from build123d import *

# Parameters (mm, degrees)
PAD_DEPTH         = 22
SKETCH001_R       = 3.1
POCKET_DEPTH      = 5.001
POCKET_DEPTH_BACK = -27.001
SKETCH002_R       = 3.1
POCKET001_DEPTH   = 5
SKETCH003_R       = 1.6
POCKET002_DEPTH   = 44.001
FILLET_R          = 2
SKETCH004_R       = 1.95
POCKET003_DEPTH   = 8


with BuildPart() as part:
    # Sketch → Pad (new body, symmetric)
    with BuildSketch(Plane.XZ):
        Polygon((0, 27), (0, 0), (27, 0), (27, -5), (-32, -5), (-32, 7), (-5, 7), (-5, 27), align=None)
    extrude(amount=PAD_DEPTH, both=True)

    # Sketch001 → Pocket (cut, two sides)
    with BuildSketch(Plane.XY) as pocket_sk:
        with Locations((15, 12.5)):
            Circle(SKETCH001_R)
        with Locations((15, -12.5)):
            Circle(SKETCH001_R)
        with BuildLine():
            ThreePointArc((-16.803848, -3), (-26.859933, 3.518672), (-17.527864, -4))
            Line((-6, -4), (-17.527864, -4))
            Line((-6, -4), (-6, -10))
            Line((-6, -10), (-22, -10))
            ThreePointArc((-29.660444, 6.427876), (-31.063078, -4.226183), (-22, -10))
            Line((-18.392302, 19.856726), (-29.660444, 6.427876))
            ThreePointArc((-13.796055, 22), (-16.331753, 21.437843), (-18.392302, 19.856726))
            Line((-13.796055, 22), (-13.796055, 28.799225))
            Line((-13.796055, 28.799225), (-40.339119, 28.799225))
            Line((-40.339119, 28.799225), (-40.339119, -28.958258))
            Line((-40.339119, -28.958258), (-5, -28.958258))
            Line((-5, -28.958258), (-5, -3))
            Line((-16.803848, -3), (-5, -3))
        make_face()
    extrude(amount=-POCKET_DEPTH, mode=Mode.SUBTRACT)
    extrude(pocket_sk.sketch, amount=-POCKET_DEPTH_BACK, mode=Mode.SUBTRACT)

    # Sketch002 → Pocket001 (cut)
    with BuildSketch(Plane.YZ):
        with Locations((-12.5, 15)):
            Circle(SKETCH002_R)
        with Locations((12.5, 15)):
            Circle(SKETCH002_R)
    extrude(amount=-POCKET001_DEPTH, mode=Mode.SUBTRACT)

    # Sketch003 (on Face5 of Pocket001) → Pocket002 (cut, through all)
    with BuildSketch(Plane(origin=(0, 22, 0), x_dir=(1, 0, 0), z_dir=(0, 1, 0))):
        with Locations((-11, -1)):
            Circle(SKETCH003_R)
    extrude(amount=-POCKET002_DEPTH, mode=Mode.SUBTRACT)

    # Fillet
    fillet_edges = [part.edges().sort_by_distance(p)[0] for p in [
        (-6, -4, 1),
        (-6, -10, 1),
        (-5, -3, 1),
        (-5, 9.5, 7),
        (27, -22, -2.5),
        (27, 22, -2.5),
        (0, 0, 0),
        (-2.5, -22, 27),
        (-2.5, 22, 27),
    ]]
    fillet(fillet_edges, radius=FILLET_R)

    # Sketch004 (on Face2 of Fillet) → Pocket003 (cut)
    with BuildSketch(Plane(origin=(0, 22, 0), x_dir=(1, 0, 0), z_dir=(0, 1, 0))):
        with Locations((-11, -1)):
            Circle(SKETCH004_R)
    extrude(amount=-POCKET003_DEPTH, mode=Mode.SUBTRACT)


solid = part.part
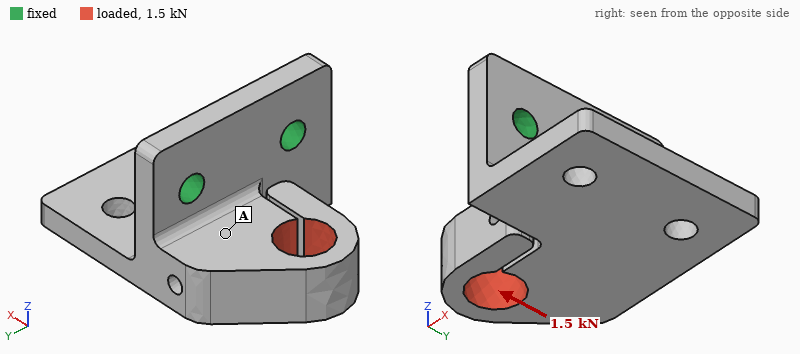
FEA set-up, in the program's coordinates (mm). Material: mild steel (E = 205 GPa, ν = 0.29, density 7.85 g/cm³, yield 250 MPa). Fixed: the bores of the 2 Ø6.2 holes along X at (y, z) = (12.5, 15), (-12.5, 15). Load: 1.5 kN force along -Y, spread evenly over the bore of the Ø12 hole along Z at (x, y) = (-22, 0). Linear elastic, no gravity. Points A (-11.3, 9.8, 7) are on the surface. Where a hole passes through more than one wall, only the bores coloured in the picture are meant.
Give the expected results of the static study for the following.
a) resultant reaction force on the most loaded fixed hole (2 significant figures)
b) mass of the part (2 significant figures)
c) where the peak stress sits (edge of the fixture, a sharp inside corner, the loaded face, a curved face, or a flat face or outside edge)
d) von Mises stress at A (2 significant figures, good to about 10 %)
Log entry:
1.4 kN
150 g
a curved face
17 MPa
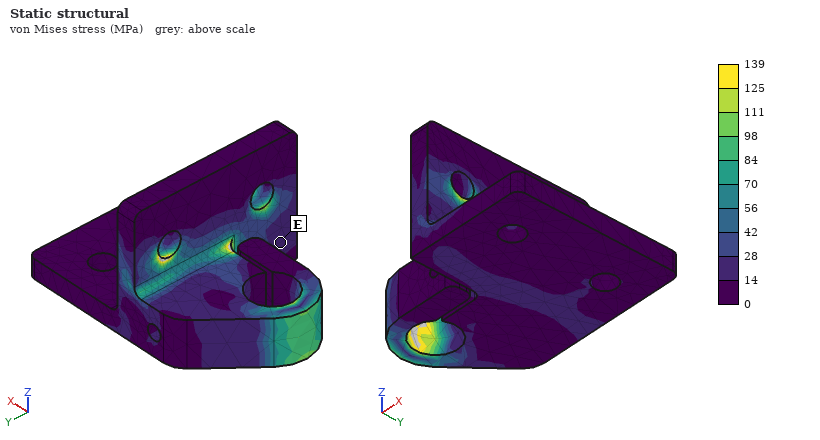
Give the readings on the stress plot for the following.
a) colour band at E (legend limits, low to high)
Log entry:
14 to 28 MPa
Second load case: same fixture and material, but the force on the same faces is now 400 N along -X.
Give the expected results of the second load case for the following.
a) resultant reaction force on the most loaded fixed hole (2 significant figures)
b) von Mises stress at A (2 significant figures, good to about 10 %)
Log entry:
210 N
3.8 MPa
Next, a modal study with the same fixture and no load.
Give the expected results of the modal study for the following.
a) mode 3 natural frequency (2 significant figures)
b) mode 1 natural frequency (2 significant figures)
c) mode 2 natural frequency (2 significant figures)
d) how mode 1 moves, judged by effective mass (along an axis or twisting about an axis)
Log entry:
3200 Hz
2300 Hz
2600 Hz
along X
